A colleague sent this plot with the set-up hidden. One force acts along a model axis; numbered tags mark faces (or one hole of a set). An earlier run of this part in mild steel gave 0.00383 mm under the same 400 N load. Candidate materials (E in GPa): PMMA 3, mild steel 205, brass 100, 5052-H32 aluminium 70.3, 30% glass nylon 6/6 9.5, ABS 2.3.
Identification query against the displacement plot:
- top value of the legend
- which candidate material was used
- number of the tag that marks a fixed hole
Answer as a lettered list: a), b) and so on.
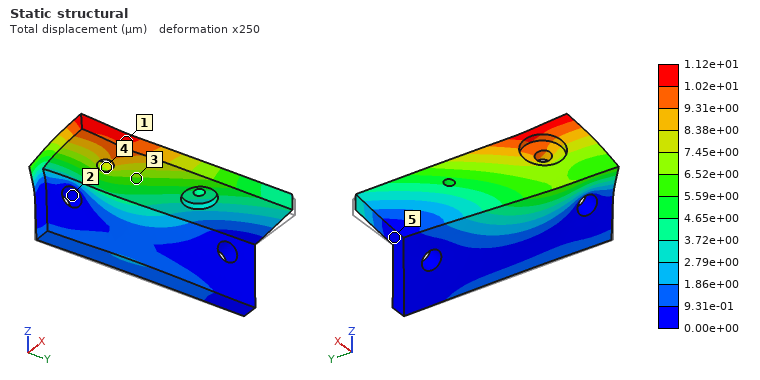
a) 1.12e+01 µm
b) 5052-H32 aluminium
c) 2
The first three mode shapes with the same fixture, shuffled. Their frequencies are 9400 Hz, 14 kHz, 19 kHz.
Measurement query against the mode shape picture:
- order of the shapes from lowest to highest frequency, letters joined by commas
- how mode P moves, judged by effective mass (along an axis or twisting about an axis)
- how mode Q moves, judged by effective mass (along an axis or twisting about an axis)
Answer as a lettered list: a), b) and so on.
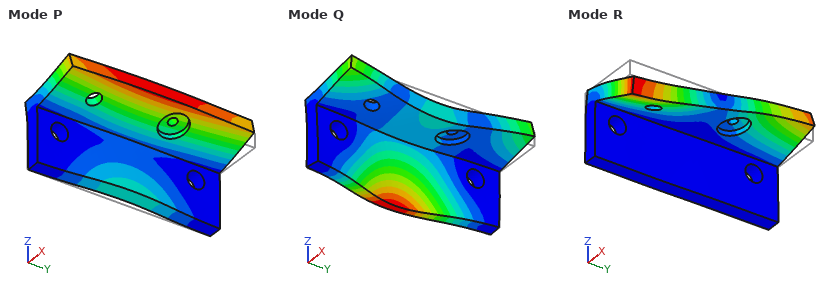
a) P, R, Q
b) along Z
c) along X
